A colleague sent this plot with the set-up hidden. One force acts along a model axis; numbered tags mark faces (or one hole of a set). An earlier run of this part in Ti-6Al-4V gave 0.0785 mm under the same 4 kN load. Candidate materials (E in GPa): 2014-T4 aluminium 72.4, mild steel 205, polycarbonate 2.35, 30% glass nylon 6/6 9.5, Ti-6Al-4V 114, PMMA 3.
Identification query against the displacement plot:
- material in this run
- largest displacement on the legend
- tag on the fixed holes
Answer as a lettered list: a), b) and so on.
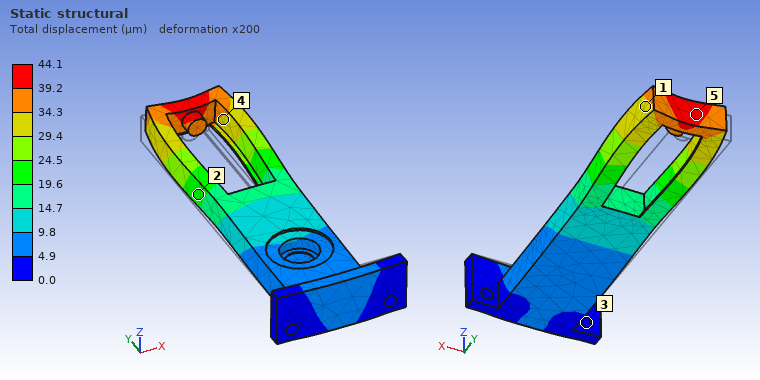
a) mild steel
b) 44.1 µm
c) 3
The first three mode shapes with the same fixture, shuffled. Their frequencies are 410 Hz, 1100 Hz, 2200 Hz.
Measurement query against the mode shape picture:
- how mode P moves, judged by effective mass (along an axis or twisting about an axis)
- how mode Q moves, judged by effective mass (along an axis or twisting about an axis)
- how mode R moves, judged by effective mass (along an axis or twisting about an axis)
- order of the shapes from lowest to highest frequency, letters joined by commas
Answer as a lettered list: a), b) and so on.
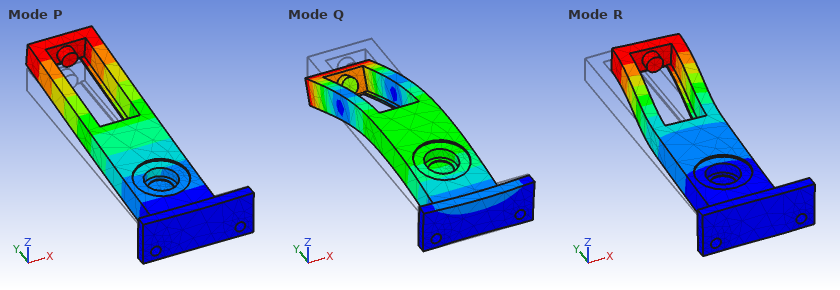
a) along Z
b) along Z
c) along X
d) P, R, Q
